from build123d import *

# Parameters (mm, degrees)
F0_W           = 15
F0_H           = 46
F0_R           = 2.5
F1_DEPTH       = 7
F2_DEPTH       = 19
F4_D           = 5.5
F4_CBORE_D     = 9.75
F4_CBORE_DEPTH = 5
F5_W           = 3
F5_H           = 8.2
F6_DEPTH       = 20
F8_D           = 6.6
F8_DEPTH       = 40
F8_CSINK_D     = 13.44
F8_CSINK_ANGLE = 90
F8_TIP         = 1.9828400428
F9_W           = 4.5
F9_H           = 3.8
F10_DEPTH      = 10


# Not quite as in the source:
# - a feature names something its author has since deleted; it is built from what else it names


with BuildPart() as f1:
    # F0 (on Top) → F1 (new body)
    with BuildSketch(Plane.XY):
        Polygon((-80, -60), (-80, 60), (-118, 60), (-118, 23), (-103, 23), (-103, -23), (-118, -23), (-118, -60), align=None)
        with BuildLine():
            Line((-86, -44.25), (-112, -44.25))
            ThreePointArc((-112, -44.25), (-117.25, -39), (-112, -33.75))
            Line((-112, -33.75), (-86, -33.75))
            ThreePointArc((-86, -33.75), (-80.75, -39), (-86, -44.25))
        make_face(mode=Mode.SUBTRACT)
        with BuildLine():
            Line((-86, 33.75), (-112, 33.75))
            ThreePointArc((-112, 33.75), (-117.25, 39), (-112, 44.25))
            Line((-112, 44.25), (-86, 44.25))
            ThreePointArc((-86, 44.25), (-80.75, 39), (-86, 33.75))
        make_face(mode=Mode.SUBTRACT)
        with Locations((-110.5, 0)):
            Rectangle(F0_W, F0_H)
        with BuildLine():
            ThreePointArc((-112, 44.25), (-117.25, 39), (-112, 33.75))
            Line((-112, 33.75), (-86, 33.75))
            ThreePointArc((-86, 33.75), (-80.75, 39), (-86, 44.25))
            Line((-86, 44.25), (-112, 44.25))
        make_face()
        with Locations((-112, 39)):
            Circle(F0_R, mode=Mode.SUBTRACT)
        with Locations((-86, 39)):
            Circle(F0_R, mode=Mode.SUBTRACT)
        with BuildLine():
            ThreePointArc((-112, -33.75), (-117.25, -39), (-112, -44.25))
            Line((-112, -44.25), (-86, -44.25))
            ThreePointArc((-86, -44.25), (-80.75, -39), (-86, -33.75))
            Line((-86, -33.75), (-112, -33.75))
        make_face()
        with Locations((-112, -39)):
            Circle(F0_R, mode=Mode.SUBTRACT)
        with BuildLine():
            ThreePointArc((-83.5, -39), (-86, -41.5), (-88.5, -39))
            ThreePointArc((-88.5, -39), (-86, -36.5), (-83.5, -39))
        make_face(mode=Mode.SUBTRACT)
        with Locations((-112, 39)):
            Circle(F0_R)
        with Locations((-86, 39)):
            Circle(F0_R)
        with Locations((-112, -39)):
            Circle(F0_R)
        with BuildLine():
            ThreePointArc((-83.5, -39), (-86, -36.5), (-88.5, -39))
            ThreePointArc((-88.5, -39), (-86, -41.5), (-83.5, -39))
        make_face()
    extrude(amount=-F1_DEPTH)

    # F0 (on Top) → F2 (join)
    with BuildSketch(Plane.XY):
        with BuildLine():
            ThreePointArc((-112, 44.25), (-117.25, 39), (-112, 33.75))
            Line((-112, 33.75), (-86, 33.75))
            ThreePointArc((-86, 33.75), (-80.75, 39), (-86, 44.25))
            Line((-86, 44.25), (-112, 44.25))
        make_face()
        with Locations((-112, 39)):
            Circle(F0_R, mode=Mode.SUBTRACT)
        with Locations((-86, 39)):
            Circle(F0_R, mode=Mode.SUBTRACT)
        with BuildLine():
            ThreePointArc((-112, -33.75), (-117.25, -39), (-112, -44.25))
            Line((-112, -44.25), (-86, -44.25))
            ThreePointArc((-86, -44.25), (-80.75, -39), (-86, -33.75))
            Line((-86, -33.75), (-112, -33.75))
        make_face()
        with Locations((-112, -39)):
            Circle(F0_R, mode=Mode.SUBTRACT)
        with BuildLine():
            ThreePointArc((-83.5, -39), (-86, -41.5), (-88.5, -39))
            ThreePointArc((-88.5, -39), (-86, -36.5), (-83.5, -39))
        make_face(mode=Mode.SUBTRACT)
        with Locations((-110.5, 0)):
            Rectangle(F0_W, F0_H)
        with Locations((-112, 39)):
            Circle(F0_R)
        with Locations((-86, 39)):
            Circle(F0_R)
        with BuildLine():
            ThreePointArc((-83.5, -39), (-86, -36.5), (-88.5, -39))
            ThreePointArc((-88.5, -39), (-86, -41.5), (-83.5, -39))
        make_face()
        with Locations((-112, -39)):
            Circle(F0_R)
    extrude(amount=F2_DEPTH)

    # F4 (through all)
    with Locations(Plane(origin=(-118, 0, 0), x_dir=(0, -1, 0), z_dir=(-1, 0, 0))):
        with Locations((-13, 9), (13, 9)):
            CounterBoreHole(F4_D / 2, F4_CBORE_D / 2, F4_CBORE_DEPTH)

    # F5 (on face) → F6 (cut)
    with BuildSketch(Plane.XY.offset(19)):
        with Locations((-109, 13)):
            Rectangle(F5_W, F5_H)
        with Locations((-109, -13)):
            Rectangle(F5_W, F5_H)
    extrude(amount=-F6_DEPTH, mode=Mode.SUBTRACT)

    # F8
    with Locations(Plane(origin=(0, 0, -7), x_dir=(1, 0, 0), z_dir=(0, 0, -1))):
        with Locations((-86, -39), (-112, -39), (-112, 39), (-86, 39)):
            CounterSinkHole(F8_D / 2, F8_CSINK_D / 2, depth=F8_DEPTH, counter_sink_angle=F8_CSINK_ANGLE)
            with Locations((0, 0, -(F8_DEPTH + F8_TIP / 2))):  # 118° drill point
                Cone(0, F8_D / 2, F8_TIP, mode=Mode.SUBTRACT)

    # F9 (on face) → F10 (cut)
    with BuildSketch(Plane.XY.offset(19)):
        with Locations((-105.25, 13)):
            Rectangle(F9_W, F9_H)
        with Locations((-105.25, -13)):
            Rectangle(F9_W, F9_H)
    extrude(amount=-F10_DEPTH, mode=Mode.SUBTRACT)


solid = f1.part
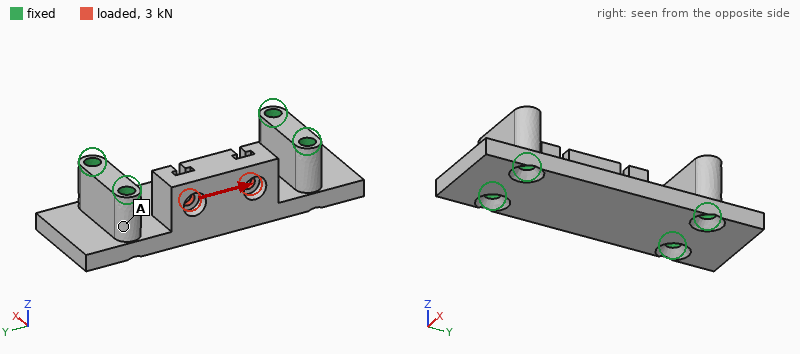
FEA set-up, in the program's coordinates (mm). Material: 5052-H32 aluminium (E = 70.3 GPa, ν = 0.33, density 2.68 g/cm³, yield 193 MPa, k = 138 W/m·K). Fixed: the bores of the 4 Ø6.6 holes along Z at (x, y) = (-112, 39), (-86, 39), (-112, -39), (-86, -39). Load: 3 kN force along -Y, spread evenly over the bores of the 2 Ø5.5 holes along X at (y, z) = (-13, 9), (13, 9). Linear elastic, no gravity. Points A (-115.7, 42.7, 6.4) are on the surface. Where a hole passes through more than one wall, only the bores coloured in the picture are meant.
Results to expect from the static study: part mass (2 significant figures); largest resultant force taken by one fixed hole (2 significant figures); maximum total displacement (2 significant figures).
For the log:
140 g
1.0 kN
18 µm
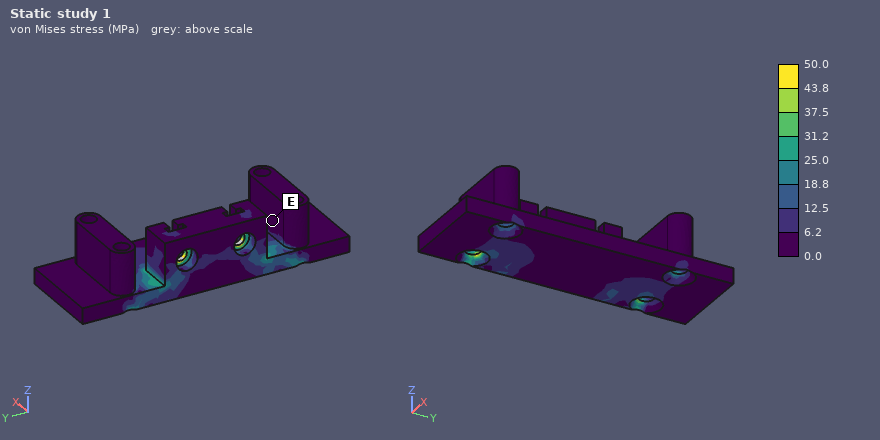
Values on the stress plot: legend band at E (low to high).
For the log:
0.0 to 6.2 MPa
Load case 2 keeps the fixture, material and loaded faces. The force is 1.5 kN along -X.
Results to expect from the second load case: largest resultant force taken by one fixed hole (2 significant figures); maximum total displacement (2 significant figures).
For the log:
590 N
45 µm
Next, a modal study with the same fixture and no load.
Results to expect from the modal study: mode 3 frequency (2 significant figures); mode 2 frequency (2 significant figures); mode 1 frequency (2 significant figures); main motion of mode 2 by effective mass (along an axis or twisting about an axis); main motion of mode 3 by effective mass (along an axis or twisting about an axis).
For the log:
11 kHz
6500 Hz
5400 Hz
along Z
along Y
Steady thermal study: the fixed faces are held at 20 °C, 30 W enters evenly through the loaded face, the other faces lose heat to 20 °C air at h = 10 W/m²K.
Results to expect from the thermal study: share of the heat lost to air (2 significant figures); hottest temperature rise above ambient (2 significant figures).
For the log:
3.2 %
21 K
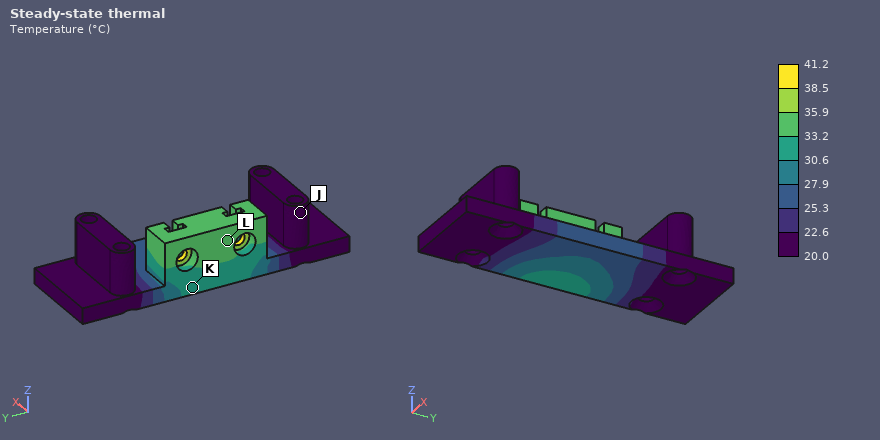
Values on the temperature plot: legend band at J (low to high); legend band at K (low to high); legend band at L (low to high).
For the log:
20.0 to 22.6 °C
30.6 to 33.2 °C
33.2 to 35.9 °C
